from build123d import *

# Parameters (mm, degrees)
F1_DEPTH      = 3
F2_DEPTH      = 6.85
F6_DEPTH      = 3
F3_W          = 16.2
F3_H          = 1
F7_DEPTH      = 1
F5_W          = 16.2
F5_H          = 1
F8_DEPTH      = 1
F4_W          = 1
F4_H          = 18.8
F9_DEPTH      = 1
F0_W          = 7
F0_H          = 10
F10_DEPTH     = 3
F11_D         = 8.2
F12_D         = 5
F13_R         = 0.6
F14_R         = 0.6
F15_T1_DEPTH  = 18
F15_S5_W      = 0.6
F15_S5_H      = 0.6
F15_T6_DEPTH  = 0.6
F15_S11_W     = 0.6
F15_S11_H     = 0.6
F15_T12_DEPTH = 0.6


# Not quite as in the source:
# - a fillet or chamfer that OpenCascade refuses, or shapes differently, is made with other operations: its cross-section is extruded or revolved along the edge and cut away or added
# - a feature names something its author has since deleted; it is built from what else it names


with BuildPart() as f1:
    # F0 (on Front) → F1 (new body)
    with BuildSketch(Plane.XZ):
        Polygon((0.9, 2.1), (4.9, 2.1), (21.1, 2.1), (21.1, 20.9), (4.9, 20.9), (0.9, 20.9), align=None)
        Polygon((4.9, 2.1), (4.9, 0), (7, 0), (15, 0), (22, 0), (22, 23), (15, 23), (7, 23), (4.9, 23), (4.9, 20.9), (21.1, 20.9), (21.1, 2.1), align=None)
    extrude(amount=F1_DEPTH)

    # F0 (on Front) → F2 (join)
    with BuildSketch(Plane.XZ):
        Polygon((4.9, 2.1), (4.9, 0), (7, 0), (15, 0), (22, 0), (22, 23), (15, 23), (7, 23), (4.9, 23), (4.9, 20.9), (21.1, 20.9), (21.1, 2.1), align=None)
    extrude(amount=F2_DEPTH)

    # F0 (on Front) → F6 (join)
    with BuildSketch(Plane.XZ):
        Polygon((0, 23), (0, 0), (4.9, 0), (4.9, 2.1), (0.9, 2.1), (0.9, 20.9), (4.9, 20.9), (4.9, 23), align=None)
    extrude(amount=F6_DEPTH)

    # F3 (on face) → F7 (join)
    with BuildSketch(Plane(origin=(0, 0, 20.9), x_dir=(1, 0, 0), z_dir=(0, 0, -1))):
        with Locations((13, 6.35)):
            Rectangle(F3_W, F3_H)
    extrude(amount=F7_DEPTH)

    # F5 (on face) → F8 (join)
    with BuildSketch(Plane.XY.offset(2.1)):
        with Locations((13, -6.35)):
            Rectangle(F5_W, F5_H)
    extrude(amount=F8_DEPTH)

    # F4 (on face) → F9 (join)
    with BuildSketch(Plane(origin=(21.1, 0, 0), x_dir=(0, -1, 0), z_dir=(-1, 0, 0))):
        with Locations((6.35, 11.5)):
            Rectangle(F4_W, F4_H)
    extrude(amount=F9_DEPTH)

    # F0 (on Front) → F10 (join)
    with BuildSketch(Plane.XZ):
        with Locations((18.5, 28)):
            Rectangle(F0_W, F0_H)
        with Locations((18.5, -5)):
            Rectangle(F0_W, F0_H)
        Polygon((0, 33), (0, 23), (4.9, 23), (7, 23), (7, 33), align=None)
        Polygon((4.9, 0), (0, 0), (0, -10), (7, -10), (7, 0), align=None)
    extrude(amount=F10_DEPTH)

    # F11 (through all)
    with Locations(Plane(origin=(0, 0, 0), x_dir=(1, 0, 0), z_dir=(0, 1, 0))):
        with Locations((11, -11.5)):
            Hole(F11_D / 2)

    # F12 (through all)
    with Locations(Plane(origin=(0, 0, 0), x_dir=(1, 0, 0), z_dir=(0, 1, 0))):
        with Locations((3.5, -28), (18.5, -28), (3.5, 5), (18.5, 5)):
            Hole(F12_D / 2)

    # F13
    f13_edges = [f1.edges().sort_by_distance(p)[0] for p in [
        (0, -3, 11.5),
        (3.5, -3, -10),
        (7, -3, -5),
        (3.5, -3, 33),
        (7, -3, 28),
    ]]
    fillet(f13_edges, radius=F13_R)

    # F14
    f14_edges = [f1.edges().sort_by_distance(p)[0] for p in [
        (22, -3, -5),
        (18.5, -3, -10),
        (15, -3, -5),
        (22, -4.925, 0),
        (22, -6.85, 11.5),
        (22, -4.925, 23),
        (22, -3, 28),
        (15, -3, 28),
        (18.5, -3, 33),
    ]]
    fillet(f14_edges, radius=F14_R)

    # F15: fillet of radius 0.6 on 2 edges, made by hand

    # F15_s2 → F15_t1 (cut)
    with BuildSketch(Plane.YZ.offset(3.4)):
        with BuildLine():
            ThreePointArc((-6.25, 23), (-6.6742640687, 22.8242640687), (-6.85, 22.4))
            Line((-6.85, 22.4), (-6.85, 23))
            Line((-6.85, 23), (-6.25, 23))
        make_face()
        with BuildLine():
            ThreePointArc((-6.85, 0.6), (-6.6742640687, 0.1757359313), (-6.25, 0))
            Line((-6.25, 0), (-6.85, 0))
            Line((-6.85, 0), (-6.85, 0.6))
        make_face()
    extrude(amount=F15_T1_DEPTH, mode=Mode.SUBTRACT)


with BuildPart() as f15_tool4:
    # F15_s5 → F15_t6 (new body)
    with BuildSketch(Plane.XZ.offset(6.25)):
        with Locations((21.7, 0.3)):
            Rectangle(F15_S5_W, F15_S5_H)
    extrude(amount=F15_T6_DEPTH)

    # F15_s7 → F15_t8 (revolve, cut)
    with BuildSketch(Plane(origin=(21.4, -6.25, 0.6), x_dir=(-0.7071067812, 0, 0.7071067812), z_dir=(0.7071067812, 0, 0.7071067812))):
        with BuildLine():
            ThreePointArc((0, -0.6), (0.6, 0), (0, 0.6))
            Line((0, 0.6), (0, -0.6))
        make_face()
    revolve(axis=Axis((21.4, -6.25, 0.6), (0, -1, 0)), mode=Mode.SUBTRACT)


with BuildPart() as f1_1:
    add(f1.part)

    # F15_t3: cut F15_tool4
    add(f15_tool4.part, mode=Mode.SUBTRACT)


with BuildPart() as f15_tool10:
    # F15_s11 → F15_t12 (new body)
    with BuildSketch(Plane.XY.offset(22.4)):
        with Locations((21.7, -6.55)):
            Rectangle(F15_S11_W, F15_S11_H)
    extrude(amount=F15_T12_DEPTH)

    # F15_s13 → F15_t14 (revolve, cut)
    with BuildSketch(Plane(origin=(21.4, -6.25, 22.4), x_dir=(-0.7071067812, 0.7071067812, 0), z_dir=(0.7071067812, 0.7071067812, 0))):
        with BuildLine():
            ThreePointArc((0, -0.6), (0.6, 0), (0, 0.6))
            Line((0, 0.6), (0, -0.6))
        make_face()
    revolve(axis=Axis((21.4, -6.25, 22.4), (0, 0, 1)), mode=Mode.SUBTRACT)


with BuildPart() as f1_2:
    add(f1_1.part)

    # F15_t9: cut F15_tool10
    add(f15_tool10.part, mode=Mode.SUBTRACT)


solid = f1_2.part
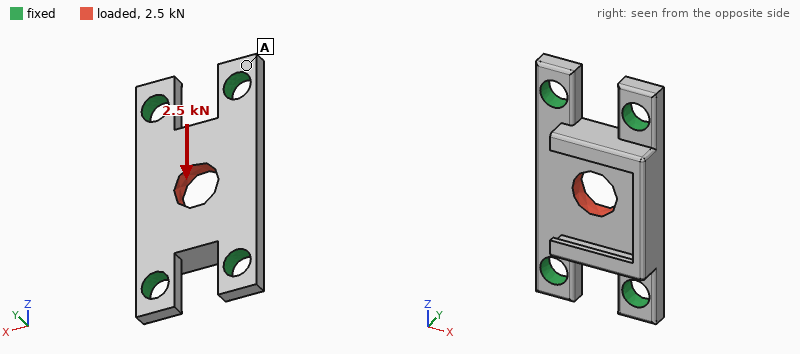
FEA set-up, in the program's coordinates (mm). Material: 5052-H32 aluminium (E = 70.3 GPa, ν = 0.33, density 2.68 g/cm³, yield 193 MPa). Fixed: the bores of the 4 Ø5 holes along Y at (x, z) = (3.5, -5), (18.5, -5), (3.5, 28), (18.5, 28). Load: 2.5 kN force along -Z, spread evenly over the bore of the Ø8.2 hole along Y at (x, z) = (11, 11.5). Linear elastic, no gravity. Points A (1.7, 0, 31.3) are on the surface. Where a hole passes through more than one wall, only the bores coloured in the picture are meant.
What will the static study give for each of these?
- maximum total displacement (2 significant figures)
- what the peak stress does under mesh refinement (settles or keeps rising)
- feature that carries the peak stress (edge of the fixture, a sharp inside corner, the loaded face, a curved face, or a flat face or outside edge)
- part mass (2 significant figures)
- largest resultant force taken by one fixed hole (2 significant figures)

6.3 µm
keeps rising
a sharp inside corner
6.3 g
650 N
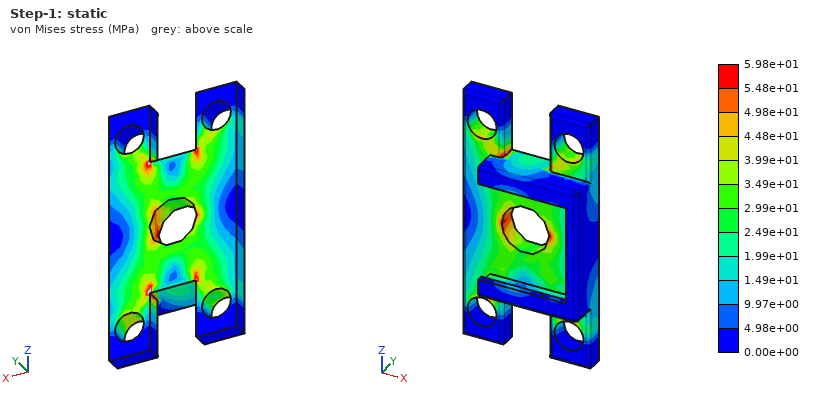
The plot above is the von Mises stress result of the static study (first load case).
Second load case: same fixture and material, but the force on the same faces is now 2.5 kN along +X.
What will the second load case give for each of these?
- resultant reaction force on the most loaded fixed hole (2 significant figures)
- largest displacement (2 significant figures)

730 N
18 µm
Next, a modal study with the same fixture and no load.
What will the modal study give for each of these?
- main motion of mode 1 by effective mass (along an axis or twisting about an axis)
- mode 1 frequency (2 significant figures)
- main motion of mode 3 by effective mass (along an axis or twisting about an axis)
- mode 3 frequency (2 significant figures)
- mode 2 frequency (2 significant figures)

along Y
17 kHz
along X
35 kHz
23 kHz
